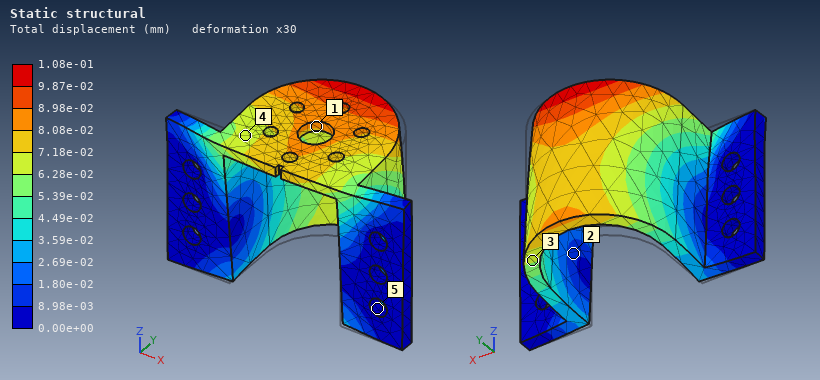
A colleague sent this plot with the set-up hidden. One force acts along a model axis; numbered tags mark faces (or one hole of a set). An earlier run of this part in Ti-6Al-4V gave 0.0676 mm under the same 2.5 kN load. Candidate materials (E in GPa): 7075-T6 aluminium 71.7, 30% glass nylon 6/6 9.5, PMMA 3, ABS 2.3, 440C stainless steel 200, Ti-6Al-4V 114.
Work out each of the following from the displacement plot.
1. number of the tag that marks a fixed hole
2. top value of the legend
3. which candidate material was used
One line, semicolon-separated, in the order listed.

5; 1.08e-01 mm; 7075-T6 aluminium
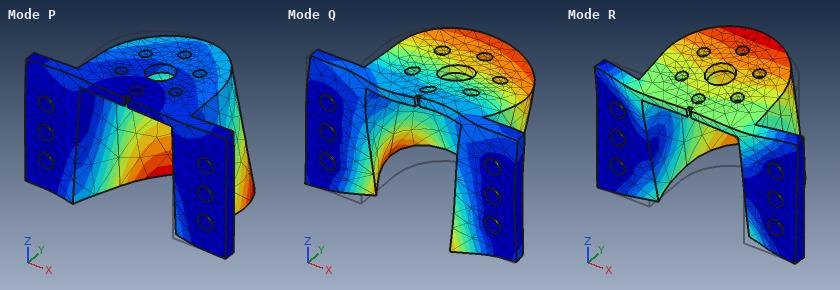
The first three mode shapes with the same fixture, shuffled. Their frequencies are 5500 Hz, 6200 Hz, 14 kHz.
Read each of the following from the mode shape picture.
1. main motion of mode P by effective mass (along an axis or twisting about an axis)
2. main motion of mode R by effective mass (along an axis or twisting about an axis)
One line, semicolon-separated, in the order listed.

along X; along Z
